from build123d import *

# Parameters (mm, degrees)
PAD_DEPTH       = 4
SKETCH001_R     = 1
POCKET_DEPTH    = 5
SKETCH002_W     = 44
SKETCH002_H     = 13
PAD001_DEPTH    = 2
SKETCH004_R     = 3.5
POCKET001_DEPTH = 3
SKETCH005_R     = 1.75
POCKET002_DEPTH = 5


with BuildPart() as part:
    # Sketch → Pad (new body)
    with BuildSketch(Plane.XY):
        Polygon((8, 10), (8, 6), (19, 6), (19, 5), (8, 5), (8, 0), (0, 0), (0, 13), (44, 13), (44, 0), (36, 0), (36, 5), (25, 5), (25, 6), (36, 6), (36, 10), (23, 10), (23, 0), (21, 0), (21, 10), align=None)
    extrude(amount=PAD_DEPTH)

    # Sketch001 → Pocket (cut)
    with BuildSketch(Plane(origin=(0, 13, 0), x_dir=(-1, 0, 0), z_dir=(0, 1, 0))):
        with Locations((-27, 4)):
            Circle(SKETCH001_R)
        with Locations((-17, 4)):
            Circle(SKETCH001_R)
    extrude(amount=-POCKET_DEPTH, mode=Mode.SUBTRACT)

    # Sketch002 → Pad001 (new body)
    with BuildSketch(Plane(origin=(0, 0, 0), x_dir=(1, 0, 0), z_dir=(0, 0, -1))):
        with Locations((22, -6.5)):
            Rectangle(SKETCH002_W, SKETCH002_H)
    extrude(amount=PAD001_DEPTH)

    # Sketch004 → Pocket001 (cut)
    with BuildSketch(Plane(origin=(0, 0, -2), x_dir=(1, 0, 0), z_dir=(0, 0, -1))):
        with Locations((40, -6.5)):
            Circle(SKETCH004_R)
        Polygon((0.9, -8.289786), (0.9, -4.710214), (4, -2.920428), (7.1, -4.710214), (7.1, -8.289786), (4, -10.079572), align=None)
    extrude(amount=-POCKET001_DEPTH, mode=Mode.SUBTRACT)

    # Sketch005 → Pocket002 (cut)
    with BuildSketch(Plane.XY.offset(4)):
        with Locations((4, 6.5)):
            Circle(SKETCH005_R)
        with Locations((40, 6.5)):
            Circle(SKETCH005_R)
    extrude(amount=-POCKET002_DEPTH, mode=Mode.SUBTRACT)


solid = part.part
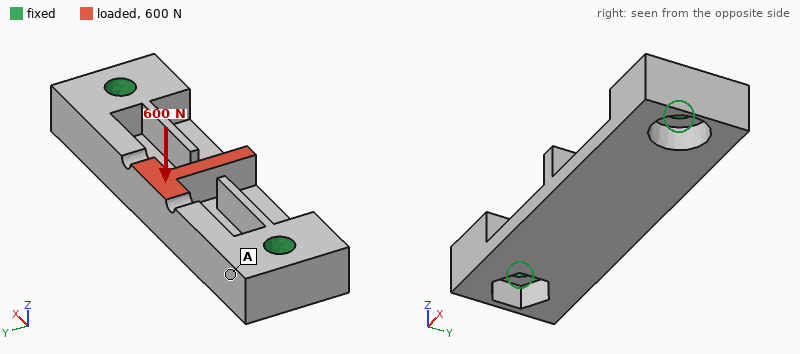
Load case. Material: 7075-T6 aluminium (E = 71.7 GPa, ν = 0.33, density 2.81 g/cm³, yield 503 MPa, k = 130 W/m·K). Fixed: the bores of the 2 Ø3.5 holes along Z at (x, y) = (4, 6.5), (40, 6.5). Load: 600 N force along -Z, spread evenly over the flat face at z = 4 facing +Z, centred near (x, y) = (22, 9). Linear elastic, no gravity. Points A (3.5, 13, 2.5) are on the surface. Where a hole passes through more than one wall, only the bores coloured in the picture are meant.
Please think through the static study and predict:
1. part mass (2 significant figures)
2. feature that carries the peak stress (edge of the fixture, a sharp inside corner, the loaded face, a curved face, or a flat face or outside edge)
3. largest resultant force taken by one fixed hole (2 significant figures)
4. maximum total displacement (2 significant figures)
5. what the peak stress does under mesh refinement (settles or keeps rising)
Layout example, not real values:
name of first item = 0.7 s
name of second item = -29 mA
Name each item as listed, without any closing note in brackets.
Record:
part mass = 6.2 g
feature that carries the peak stress = edge of the fixture
largest resultant force taken by one fixed hole = 530 N
maximum total displacement = 40 µm
what the peak stress does under mesh refinement = keeps rising
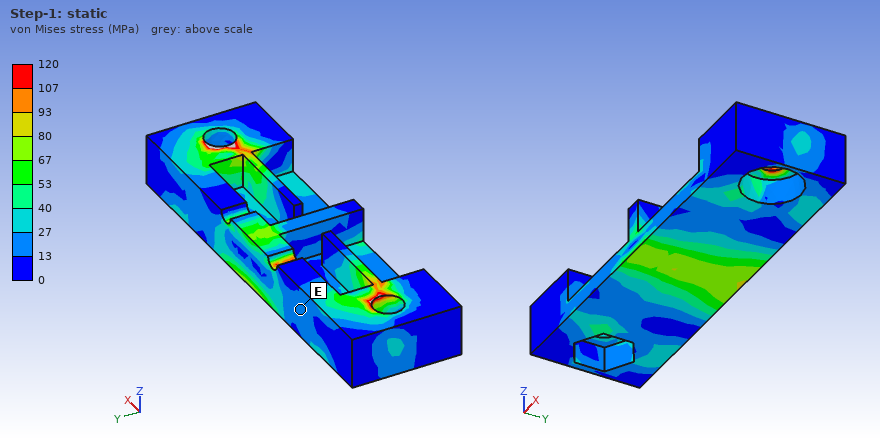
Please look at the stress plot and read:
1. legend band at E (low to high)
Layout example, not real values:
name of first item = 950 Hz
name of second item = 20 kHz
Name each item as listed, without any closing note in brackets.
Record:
legend band at E = 13 to 27 MPa
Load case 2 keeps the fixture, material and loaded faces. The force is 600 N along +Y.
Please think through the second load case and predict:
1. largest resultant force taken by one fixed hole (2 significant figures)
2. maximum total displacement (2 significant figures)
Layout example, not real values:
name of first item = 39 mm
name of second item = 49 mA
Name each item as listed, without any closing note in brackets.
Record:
largest resultant force taken by one fixed hole = 300 N
maximum total displacement = 72 µm
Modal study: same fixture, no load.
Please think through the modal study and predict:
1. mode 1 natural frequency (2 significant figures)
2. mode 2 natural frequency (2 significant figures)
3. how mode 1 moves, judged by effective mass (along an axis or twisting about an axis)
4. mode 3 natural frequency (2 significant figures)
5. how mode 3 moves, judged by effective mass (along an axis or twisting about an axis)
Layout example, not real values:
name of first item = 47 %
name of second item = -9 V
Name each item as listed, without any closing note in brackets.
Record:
mode 1 natural frequency = 15 kHz
mode 2 natural frequency = 18 kHz
how mode 1 moves, judged by effective mass = along Z
mode 3 natural frequency = 20 kHz
how mode 3 moves, judged by effective mass = along Y
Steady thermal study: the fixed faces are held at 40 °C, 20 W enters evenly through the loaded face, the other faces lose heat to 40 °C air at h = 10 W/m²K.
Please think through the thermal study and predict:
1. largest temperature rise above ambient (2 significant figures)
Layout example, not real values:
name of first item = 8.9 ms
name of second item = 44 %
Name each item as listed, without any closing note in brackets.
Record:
largest temperature rise above ambient = 47 K
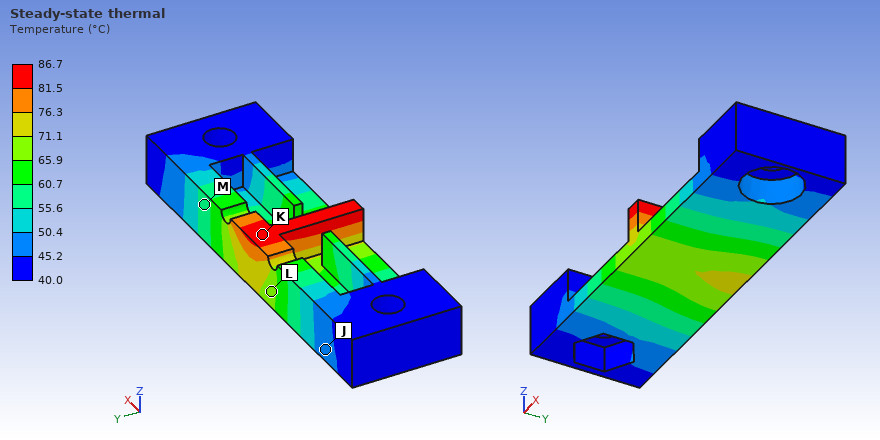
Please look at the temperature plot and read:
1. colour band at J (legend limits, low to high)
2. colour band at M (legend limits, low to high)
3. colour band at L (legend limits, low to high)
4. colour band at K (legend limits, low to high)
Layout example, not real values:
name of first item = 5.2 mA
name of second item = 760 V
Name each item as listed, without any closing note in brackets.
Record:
colour band at J = 45.2 to 50.4 °C
colour band at M = 55.6 to 60.7 °C
colour band at L = 65.9 to 71.1 °C
colour band at K = 81.5 to 86.7 °C
